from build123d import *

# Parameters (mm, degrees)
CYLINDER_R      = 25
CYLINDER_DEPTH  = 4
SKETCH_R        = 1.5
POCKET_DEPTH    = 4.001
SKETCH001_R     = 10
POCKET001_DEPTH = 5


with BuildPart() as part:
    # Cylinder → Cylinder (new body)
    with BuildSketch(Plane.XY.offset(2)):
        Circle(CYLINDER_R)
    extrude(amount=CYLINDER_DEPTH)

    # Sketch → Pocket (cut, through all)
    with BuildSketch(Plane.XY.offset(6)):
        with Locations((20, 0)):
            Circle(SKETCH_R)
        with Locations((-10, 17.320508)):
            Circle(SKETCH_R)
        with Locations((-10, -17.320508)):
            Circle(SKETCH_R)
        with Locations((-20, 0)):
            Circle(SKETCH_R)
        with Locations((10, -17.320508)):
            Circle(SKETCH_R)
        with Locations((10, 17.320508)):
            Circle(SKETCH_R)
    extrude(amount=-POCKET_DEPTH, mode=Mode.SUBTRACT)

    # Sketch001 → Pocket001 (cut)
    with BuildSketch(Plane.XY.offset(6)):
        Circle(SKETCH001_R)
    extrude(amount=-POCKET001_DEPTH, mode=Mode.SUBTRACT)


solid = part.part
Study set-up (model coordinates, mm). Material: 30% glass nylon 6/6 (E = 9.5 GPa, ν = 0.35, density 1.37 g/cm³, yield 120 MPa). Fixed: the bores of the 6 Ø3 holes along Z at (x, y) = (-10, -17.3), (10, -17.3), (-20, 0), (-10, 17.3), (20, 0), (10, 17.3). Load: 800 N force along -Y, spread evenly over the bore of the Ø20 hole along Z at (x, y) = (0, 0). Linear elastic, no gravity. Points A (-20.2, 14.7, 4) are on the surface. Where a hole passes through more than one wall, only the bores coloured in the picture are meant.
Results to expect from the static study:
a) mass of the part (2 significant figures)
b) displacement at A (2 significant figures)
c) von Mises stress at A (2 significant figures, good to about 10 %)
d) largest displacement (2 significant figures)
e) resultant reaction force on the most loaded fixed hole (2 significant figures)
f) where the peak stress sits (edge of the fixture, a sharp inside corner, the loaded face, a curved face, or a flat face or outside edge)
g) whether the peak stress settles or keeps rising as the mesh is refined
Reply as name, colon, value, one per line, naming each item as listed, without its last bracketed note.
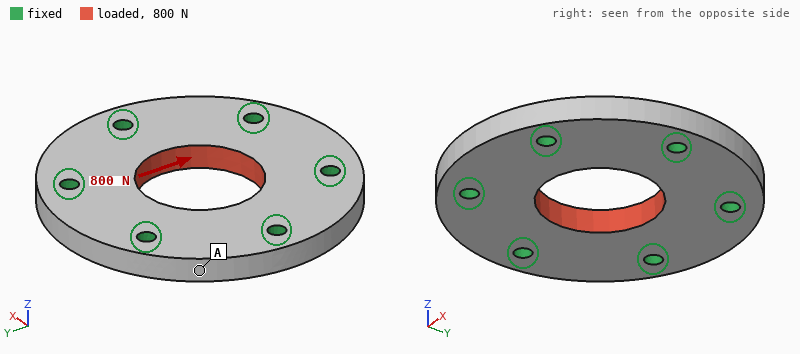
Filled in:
mass of the part: 8.8 g
displacement at A: 1.7 µm
von Mises stress at A: 1.2 MPa
largest displacement: 5.4 µm
resultant reaction force on the most loaded fixed hole: 170 N
where the peak stress sits: edge of the fixture
whether the peak stress settles or keeps rising as the mesh is refined: keeps rising
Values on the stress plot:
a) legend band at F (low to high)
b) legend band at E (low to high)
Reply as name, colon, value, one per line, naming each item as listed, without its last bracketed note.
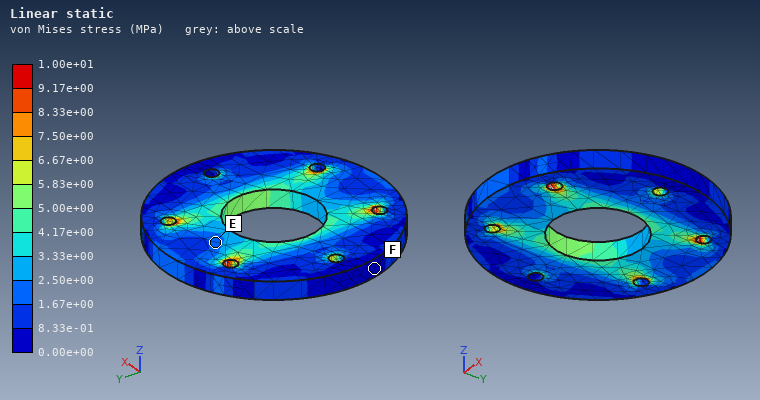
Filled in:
legend band at F: 0.00e+00 to 8.33e-01 MPa
legend band at E: 1.67e+00 to 2.50e+00 MPa
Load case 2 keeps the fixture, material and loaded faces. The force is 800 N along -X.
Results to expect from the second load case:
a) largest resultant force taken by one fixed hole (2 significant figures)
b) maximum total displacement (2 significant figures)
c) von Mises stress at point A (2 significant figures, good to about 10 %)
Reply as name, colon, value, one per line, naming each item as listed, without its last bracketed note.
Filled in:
largest resultant force taken by one fixed hole: 190 N
maximum total displacement: 5.4 µm
von Mises stress at point A: 1.8 MPa
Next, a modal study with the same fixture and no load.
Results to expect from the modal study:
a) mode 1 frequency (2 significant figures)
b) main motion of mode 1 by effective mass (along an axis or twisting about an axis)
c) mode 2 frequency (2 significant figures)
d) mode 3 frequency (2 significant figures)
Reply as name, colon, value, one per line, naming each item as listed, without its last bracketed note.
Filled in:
mode 1 frequency: 15 kHz
main motion of mode 1 by effective mass: along Z
mode 2 frequency: 18 kHz
mode 3 frequency: 19 kHz
